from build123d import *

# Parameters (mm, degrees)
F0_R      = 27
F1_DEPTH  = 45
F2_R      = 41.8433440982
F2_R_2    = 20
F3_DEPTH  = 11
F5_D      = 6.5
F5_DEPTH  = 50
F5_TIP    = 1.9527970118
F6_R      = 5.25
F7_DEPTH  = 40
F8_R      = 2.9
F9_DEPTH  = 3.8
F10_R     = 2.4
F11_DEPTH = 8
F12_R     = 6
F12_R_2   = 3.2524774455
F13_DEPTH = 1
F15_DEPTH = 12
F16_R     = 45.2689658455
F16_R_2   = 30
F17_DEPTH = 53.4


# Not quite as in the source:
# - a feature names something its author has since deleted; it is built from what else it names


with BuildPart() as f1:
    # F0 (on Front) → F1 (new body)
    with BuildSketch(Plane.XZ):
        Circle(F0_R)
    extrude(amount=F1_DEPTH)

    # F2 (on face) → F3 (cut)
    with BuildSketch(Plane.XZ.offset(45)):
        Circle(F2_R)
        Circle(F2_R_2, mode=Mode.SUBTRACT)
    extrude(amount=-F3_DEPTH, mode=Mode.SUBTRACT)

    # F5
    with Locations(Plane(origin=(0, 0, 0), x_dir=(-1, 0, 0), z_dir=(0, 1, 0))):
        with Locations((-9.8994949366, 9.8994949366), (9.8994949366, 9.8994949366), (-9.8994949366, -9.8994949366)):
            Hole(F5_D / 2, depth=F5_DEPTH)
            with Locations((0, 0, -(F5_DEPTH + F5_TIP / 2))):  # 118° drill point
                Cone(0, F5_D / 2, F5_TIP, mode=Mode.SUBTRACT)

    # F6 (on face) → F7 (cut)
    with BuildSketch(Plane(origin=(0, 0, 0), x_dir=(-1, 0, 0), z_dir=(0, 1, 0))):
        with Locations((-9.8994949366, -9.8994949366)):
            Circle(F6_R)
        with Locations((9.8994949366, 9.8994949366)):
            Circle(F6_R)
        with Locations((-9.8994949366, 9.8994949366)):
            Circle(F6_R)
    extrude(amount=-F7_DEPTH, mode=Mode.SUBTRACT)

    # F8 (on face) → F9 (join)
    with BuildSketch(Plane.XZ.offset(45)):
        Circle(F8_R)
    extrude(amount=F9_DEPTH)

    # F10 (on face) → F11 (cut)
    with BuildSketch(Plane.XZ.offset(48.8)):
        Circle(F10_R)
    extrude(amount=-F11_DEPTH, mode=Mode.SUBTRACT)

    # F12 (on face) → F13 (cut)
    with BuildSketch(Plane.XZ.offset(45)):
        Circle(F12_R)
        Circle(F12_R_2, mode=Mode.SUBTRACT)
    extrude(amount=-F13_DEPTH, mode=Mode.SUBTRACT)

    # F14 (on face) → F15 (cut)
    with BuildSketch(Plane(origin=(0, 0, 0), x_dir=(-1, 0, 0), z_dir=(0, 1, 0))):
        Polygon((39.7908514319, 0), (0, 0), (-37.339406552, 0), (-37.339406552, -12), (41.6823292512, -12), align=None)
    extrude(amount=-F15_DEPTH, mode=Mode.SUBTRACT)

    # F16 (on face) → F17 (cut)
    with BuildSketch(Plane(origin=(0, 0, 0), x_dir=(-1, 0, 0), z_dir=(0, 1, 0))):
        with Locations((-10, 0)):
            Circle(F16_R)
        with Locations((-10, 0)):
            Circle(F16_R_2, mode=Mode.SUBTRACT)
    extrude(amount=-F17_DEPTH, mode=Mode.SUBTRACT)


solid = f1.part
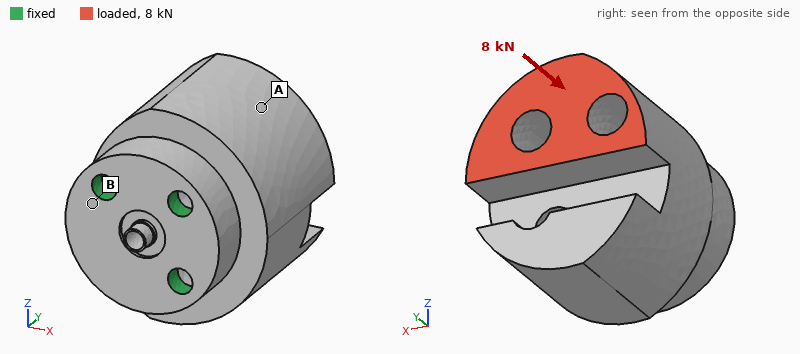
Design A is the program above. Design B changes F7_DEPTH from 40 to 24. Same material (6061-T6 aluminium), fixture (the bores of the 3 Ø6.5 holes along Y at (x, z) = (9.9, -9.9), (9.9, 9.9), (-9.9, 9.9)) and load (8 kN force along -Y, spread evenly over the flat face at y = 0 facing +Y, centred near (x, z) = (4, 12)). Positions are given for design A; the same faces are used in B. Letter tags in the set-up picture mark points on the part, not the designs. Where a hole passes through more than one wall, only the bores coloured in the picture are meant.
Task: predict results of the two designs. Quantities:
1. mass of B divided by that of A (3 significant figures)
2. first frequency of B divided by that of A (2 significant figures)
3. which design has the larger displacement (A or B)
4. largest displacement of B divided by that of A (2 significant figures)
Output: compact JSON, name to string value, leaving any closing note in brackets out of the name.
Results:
{"mass of B divided by that of A": "1.04", "first frequency of B divided by that of A": "3.1", "which design has the larger displacement": "A", "largest displacement of B divided by that of A": "0.25"}
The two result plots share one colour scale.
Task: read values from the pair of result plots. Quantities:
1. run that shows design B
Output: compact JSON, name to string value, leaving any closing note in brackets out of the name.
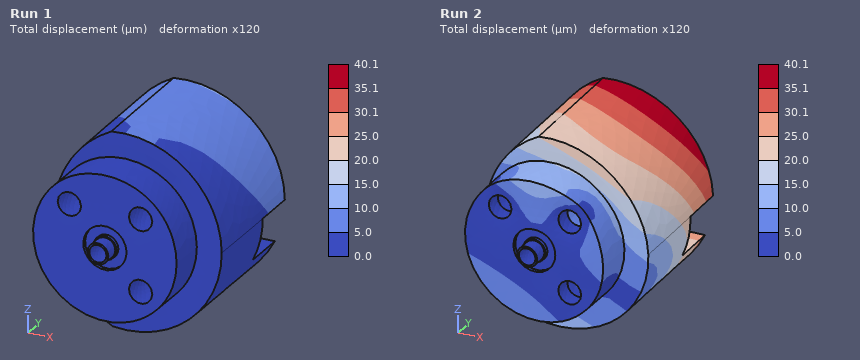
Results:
{"run that shows design B": "Run 1"}
